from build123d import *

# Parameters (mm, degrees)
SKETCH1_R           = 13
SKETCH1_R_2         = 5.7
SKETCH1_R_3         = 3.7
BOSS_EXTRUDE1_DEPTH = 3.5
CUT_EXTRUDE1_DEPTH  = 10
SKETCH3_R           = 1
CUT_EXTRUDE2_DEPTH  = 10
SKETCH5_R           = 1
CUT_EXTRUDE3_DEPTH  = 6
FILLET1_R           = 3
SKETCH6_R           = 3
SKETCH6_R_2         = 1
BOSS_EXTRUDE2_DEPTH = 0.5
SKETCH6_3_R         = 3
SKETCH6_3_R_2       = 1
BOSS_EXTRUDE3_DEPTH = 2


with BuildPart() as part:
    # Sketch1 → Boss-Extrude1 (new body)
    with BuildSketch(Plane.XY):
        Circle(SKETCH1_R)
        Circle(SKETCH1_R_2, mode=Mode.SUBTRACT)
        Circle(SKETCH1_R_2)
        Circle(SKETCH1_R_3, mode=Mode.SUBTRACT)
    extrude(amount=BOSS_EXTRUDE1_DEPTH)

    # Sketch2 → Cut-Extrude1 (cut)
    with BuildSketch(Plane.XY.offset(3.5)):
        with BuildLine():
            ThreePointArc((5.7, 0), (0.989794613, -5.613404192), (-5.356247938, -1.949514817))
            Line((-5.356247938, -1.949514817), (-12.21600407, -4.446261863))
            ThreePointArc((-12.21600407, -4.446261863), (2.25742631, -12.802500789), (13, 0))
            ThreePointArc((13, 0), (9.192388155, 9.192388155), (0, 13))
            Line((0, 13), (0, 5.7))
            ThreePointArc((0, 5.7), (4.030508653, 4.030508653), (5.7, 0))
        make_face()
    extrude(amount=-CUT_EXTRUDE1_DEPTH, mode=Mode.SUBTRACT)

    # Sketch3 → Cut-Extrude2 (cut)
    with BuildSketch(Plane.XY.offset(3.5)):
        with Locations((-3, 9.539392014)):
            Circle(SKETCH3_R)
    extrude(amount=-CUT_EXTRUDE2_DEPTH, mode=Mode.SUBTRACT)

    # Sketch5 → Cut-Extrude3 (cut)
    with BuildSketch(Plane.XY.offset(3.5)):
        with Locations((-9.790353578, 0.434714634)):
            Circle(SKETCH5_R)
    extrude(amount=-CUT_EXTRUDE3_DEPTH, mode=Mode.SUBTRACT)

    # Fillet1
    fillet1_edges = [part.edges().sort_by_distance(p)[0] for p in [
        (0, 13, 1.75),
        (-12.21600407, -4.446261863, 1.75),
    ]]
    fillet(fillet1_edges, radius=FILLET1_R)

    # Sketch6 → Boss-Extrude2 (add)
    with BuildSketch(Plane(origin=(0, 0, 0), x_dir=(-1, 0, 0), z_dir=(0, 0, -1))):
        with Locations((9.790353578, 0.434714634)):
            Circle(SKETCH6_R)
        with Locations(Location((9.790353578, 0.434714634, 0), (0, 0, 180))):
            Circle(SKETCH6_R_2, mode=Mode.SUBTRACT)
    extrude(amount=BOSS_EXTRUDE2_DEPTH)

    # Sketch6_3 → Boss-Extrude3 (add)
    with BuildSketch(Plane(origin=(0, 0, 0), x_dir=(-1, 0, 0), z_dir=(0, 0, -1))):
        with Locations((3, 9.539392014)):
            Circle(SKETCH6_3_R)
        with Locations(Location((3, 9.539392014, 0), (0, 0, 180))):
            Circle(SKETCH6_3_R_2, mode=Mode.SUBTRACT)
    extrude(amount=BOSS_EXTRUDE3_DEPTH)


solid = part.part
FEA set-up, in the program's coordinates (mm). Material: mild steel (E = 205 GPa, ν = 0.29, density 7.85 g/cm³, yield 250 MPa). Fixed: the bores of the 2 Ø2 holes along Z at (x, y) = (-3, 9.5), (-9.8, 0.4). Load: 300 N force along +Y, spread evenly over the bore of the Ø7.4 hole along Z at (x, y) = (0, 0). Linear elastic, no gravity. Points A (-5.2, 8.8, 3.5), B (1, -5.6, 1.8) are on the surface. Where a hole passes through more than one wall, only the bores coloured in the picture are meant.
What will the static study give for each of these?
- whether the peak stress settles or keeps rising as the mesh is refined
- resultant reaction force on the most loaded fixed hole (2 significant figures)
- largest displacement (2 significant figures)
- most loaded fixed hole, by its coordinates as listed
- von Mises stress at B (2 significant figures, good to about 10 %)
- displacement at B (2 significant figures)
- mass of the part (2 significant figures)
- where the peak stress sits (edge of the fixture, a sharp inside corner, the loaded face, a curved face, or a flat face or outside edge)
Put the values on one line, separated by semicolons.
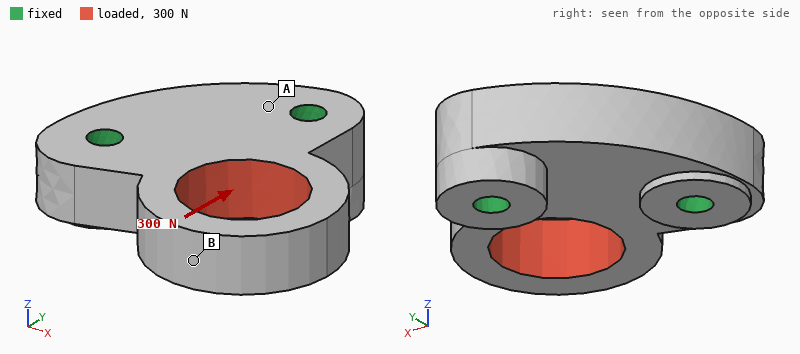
keeps rising; 280 N; 7.1 µm; (-3, 9.5); 39 MPa; 6.8 µm; 5.4 g; a sharp inside corner
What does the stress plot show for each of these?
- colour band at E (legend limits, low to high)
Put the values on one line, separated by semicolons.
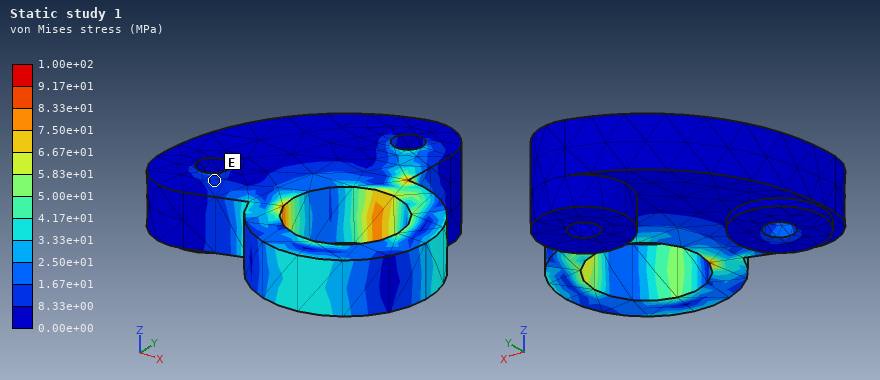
8.33e+00 to 1.67e+01 MPa
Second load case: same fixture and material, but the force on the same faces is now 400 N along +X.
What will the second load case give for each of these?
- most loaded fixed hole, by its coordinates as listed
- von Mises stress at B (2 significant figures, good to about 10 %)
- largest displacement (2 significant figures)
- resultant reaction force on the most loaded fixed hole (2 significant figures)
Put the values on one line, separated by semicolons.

(-9.8, 0.4); 31 MPa; 6.8 µm; 350 N
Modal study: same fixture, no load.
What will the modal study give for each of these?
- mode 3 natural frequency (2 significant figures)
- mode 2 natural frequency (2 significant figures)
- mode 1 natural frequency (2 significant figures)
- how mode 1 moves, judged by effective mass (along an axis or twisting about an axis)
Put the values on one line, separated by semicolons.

39 kHz; 25 kHz; 17 kHz; along Z
